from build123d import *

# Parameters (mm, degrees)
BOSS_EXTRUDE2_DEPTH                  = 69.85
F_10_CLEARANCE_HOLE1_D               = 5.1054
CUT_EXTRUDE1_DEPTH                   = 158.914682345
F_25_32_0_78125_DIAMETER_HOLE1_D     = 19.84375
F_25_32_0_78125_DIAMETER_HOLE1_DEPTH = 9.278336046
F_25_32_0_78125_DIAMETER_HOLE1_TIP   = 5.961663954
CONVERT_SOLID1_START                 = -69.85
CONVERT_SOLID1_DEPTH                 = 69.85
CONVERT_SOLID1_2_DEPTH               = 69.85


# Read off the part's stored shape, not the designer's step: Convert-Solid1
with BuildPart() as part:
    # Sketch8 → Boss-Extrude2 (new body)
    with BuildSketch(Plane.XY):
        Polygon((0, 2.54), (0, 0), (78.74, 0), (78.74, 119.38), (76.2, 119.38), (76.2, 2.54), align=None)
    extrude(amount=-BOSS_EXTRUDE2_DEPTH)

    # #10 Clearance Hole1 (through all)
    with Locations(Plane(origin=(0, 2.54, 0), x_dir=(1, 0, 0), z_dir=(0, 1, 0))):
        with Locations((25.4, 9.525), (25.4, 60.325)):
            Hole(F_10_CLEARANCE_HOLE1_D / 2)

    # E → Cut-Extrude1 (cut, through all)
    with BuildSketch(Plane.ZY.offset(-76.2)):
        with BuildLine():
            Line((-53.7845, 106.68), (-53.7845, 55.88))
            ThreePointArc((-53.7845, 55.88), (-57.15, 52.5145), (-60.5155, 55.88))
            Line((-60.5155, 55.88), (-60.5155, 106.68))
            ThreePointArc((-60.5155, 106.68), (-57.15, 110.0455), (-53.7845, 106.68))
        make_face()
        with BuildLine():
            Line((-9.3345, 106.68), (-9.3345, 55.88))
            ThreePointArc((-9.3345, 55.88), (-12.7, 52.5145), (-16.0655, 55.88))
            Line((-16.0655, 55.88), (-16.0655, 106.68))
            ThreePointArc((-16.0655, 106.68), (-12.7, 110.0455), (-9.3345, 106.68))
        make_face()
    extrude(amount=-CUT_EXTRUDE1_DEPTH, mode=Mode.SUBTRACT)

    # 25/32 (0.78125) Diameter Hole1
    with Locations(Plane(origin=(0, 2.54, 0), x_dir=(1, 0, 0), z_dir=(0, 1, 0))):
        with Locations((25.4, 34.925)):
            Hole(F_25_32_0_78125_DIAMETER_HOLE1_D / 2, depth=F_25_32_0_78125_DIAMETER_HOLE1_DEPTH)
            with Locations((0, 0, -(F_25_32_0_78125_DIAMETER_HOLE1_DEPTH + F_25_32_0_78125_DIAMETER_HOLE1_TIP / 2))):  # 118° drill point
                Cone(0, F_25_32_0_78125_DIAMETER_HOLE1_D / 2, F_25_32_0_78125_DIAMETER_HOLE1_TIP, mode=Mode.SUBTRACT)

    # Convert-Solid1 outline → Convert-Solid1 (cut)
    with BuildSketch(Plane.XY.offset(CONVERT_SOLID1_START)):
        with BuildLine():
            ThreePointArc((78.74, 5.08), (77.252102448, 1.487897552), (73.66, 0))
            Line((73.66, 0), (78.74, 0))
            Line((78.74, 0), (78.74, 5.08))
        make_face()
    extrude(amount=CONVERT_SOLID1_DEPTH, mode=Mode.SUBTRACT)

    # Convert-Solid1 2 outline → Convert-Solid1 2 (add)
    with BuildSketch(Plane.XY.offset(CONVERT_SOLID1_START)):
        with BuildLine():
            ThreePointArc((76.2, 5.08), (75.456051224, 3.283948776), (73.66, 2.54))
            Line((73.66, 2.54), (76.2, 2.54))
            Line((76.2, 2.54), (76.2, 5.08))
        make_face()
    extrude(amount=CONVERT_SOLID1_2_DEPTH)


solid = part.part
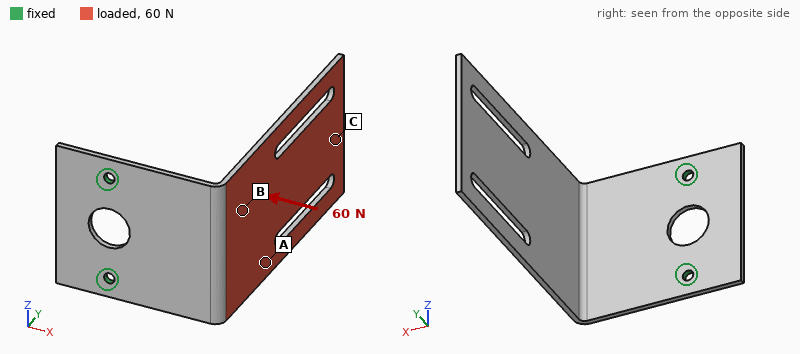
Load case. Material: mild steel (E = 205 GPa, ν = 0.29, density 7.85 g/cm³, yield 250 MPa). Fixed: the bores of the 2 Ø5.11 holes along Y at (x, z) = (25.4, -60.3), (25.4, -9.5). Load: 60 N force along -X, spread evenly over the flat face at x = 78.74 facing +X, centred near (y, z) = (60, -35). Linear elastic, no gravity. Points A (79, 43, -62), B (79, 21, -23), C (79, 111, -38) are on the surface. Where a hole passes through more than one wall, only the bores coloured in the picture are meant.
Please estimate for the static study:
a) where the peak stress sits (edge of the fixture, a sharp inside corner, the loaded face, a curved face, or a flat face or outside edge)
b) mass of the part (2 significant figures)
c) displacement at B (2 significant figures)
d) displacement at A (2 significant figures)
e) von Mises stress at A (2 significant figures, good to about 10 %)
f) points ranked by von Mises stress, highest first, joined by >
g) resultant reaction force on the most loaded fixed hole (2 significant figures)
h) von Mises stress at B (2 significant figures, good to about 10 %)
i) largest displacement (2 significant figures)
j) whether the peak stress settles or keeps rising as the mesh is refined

edge of the fixture
250 g
0.36 mm
0.59 mm
19 MPa
B > A > C
32 N
29 MPa
1.7 mm
keeps rising
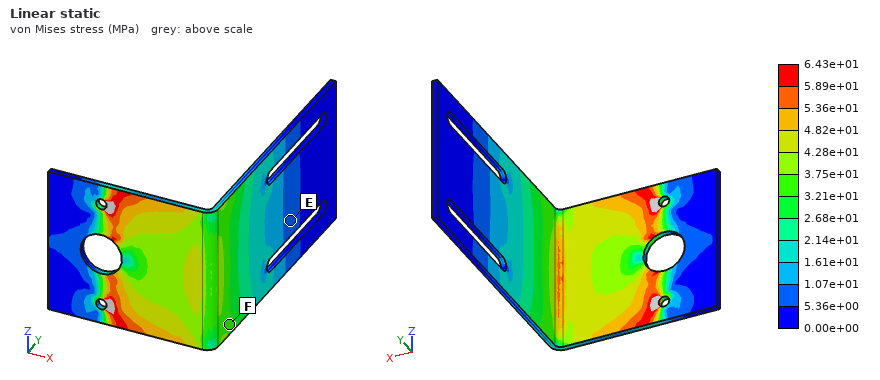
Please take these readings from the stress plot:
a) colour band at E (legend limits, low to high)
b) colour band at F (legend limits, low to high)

5.36e+00 to 1.07e+01 MPa
3.21e+01 to 3.75e+01 MPa
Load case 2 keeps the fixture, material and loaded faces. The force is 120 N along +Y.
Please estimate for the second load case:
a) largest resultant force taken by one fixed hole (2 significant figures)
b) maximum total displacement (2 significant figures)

60 N
1.2 mm
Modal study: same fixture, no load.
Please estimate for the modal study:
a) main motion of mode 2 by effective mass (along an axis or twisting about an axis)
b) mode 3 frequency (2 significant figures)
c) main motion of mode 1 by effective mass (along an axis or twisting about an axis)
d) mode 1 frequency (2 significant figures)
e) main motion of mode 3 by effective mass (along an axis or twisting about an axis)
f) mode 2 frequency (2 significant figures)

along Z
340 Hz
along X
93 Hz
along Y
190 Hz
